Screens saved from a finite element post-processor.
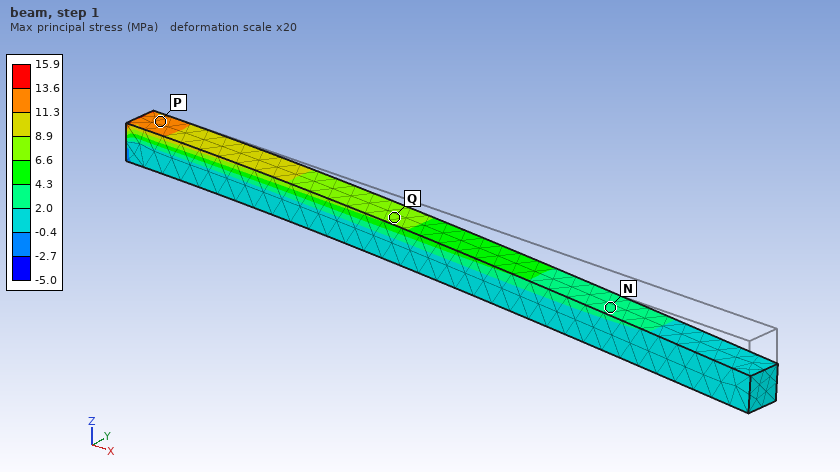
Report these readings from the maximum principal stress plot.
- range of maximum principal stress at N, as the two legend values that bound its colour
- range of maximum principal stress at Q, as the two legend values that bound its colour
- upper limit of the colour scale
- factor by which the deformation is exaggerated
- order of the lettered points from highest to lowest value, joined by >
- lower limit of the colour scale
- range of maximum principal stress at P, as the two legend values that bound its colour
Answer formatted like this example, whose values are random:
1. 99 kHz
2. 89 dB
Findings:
1. 2.0 to 4.3 MPa
2. 6.6 to 8.9 MPa
3. 15.9 MPa
4. 20
5. P > Q > N
6. -5.0 MPa
7. 11.3 to 13.6 MPa
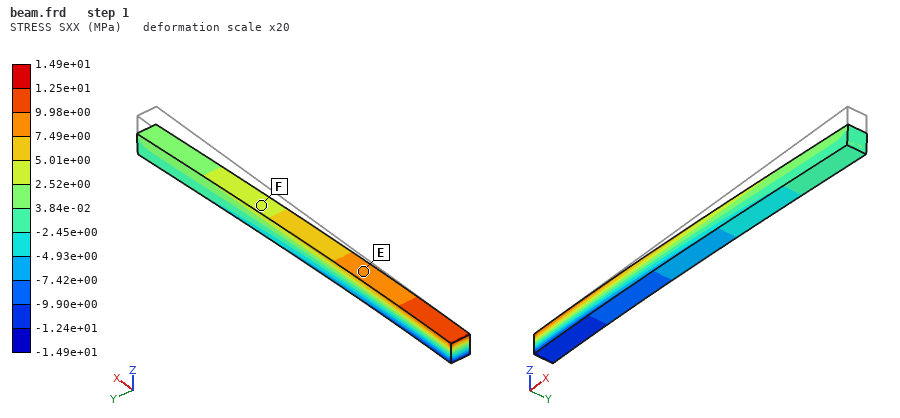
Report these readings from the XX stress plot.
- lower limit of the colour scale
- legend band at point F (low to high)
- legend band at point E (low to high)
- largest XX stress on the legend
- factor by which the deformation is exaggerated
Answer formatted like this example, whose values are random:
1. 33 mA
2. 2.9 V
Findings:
1. -1.49e+01 MPa
2. 2.52e+00 to 5.01e+00 MPa
3. 7.49e+00 to 9.98e+00 MPa
4. 1.49e+01 MPa
5. 20
